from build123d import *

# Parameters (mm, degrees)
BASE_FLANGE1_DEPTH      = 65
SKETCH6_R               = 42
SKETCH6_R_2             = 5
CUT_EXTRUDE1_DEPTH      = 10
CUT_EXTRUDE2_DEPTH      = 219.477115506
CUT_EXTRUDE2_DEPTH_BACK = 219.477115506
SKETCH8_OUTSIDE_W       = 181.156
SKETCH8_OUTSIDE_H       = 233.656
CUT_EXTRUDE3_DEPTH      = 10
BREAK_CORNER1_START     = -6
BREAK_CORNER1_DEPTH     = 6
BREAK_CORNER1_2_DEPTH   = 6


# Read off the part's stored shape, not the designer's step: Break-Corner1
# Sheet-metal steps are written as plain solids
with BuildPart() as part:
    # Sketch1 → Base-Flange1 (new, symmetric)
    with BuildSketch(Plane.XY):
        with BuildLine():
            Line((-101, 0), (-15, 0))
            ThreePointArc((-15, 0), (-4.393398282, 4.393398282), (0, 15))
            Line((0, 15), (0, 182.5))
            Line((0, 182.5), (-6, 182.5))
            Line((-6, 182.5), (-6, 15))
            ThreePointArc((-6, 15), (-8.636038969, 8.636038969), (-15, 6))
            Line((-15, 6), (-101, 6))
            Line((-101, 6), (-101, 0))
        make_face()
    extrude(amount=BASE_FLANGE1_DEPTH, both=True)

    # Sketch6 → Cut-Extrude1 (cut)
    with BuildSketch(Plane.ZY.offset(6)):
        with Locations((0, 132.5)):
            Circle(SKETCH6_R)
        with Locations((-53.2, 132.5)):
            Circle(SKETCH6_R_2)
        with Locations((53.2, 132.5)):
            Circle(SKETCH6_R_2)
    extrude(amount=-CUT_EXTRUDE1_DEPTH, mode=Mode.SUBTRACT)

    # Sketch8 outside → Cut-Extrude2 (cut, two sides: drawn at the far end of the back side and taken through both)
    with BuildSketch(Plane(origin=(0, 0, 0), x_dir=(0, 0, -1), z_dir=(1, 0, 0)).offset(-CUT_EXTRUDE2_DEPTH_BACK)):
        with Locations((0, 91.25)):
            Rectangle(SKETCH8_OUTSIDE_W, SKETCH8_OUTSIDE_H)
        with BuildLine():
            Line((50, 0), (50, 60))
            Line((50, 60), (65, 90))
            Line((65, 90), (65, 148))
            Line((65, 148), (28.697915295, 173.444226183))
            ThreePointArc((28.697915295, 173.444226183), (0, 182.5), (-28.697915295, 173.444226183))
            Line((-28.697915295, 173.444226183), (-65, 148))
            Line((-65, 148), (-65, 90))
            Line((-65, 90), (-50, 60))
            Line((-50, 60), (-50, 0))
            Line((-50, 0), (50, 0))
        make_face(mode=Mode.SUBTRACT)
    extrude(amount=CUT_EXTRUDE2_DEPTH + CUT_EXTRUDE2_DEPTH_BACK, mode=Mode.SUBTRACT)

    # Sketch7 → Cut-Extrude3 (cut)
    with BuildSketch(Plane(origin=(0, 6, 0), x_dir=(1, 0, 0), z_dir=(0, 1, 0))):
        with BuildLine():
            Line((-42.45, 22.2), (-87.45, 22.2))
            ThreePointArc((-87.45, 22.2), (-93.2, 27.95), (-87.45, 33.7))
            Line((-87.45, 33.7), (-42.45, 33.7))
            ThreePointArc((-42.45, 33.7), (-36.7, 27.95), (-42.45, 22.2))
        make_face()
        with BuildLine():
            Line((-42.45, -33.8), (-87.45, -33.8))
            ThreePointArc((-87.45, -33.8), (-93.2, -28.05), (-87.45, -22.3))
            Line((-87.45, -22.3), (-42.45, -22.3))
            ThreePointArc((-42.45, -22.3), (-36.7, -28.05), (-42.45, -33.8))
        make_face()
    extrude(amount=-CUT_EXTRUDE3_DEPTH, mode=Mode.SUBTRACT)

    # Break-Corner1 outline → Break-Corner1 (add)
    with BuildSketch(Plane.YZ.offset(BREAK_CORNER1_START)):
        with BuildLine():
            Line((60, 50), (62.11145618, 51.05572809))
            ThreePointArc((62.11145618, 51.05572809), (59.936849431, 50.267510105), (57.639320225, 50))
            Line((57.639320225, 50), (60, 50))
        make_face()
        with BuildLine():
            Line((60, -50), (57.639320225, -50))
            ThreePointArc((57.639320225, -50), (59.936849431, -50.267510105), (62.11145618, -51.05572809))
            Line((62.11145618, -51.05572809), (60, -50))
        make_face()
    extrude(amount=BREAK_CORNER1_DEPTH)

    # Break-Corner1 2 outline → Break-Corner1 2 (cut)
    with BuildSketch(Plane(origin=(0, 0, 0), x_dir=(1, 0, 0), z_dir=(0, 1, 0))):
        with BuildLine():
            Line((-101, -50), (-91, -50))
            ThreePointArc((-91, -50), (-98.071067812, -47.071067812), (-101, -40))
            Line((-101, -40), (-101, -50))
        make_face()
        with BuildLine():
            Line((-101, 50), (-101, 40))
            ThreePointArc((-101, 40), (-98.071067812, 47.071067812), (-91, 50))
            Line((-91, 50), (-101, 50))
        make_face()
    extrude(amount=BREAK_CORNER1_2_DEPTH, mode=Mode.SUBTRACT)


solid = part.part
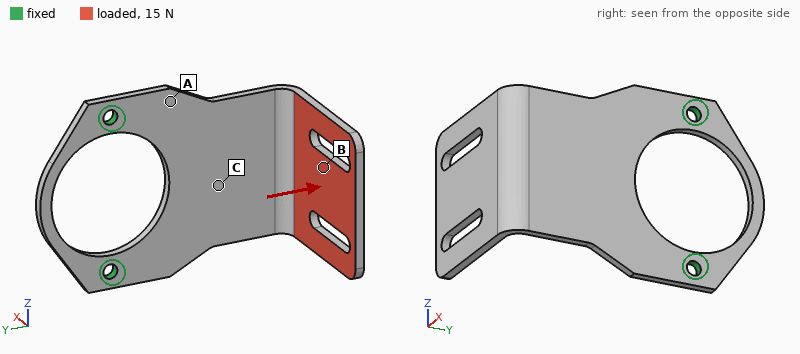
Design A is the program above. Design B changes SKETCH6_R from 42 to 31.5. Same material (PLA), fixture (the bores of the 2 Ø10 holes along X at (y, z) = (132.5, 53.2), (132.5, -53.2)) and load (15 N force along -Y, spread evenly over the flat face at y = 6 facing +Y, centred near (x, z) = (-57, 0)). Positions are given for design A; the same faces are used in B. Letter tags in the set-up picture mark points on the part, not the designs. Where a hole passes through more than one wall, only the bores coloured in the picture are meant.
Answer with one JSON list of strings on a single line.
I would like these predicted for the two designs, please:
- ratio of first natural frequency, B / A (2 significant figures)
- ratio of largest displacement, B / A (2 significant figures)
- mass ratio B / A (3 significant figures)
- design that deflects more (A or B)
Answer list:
["1.1", "0.84", "1.11", "A"]
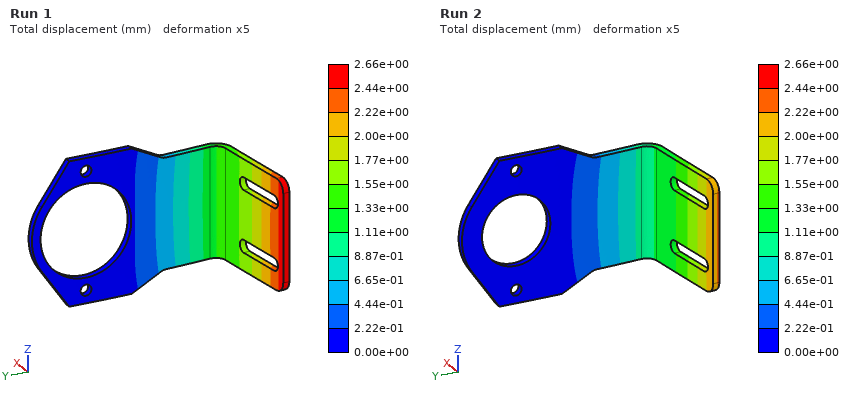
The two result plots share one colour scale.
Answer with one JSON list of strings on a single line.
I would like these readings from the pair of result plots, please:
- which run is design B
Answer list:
["Run 2"]
